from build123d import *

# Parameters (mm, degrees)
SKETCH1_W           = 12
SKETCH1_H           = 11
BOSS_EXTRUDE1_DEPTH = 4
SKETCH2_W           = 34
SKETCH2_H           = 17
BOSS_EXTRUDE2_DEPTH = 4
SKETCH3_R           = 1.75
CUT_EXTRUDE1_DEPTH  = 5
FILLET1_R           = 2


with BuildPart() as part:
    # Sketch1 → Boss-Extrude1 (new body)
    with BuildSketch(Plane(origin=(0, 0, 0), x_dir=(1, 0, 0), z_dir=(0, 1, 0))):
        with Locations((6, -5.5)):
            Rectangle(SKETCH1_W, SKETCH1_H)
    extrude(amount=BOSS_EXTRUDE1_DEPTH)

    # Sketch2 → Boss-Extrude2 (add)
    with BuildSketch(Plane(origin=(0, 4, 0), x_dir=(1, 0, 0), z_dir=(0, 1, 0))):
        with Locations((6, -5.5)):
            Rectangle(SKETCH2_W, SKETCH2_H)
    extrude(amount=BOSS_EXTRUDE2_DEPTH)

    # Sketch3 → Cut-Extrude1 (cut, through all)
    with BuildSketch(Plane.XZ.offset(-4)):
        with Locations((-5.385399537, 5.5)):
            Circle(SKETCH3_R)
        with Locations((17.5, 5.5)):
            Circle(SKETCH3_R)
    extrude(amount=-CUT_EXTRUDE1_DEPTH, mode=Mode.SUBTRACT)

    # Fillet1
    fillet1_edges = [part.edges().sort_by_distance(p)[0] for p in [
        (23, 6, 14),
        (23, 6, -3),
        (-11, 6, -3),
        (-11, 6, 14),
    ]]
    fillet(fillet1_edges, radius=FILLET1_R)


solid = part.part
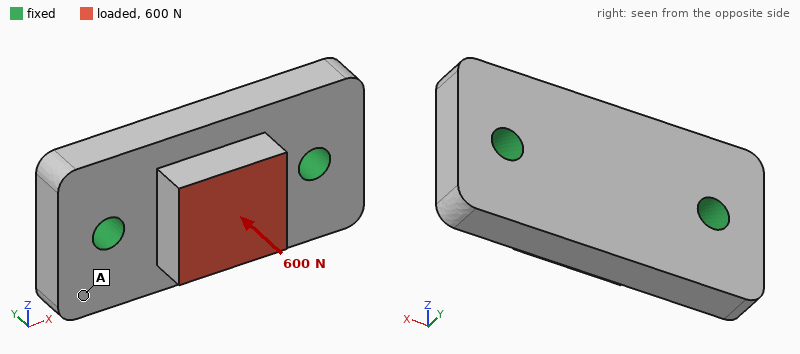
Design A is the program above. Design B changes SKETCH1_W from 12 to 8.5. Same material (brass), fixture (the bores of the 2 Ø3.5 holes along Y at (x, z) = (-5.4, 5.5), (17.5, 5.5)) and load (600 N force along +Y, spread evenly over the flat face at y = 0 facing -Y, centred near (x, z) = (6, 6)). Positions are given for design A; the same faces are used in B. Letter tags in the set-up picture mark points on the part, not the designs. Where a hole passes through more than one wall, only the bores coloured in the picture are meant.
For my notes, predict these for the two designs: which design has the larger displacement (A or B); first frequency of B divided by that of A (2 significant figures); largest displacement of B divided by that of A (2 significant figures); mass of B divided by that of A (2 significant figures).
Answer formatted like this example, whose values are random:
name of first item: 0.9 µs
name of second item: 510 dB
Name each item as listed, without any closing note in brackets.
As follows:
which design has the larger displacement: B
first frequency of B divided by that of A: 1.0
largest displacement of B divided by that of A: 1.3
mass of B divided by that of A: 0.94
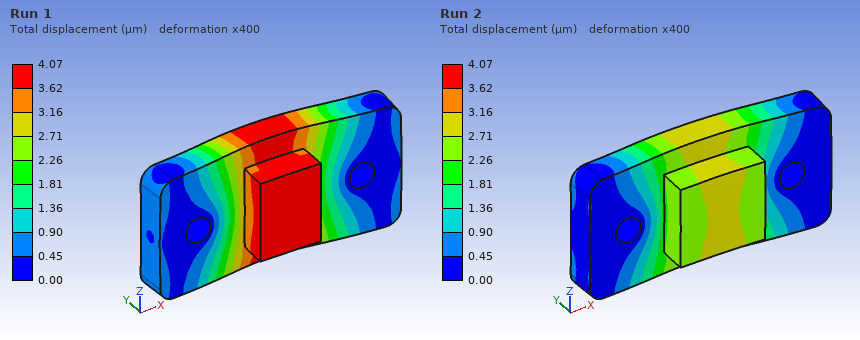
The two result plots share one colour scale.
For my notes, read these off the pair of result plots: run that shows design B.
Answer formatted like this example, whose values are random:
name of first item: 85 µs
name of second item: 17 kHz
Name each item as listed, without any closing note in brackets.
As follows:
run that shows design B: Run 1
